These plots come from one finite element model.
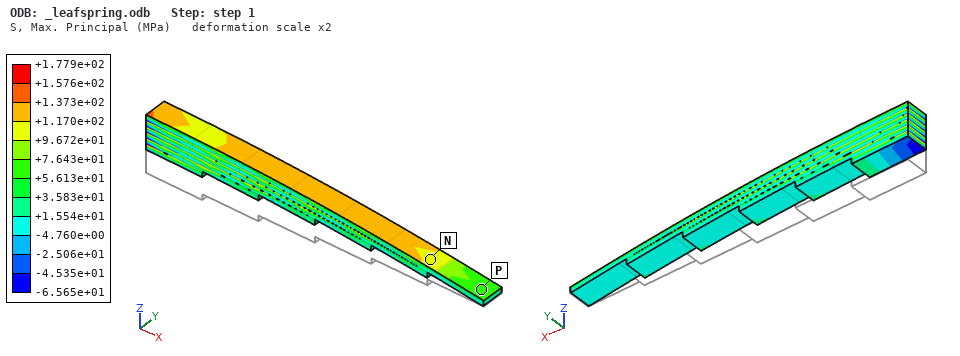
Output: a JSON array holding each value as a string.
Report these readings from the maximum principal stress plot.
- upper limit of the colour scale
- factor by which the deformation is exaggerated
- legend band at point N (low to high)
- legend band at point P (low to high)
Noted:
["+1.779e+02 MPa", "2", "+9.672e+01 to +1.170e+02 MPa", "+5.613e+01 to +7.643e+01 MPa"]
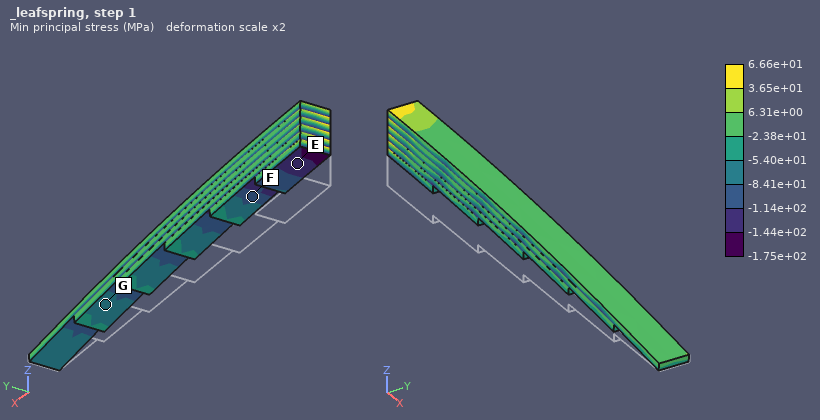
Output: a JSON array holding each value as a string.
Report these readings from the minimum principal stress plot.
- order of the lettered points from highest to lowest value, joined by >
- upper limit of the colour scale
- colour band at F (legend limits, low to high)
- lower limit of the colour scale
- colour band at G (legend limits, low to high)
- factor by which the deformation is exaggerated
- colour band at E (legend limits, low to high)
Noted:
["G > F > E", "6.66e+01 MPa", "-1.14e+02 to -8.41e+01 MPa", "-1.75e+02 MPa", "-8.41e+01 to -5.40e+01 MPa", "2", "-1.44e+02 to -1.14e+02 MPa"]
